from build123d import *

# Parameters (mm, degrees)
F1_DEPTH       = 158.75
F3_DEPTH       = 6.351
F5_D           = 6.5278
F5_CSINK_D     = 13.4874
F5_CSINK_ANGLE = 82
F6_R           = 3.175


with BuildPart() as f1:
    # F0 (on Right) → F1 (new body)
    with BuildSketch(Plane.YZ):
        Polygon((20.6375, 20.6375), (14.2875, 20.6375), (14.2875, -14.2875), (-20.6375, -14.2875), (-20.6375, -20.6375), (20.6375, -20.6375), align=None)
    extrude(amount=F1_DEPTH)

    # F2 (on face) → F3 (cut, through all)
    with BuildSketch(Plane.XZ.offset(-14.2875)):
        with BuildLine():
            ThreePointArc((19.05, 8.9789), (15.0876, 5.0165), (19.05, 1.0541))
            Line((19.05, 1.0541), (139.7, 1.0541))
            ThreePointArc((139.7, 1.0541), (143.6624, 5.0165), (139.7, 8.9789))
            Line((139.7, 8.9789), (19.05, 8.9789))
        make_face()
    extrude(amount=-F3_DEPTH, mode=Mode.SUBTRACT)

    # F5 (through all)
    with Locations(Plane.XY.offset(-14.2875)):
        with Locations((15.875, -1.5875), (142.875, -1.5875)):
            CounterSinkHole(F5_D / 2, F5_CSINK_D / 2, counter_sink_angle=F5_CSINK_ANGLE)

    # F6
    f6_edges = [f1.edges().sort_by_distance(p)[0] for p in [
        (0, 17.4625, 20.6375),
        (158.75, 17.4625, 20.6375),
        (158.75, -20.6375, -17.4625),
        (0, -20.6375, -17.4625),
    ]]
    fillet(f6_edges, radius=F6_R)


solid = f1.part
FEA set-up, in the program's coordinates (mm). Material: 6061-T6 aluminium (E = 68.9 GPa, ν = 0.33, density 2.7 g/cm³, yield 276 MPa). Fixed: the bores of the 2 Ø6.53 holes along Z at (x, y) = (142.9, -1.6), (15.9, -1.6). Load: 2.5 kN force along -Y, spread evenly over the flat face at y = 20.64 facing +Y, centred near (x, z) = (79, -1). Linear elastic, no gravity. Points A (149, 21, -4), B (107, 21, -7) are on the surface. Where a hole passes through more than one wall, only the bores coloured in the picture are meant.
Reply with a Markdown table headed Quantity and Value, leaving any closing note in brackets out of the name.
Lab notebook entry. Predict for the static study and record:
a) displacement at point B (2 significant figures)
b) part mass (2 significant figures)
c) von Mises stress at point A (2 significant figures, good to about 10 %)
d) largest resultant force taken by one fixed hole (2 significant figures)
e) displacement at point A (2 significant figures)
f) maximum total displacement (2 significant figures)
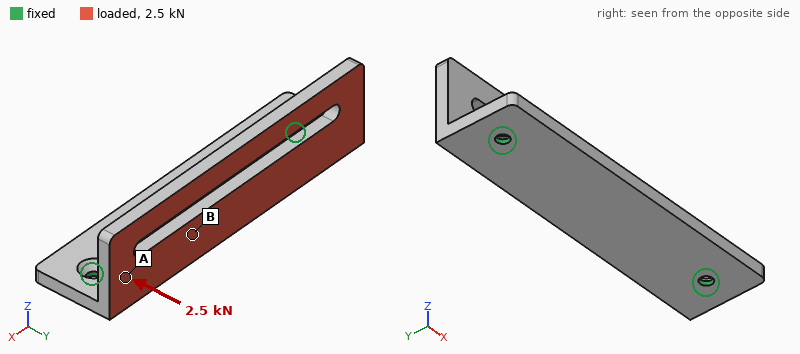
| Quantity | Value |
|---|---|
| displacement at point B | 0.25 mm |
| part mass | 190 g |
| von Mises stress at point A | 67 MPa |
| largest resultant force taken by one fixed hole | 1.3 kN |
| displacement at point A | 0.28 mm |
| maximum total displacement | 1.1 mm |
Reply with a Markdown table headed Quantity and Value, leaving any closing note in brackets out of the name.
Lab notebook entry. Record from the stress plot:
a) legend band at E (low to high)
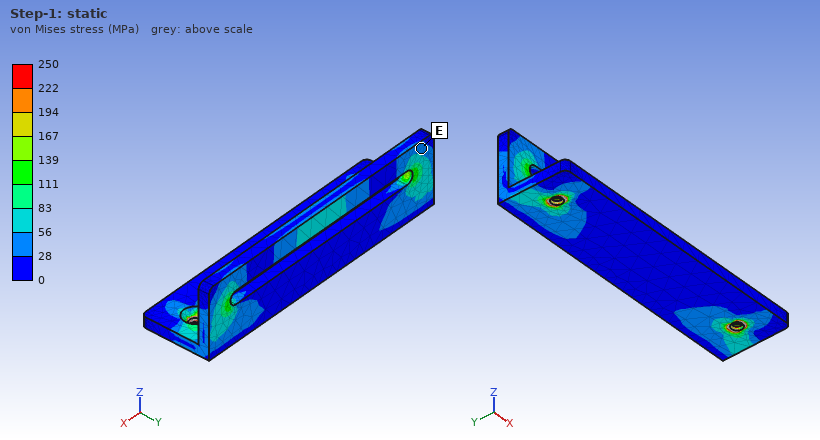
| Quantity | Value |
|---|---|
| legend band at E | 28 to 56 MPa |
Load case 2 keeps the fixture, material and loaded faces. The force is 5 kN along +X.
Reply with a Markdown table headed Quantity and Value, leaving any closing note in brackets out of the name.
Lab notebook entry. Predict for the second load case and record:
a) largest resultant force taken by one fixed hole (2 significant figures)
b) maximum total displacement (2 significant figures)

| Quantity | Value |
|---|---|
| largest resultant force taken by one fixed hole | 2.7 kN |
| maximum total displacement | 0.12 mm |
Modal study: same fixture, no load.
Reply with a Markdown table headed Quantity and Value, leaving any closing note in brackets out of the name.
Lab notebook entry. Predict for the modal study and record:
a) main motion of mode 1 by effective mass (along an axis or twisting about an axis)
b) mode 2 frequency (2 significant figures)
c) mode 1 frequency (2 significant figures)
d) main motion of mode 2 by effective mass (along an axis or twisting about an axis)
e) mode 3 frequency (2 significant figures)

| Quantity | Value |
|---|---|
| main motion of mode 1 by effective mass | along Y |
| mode 2 frequency | 1800 Hz |
| mode 1 frequency | 940 Hz |
| main motion of mode 2 by effective mass | along Z |
| mode 3 frequency | 1900 Hz |
